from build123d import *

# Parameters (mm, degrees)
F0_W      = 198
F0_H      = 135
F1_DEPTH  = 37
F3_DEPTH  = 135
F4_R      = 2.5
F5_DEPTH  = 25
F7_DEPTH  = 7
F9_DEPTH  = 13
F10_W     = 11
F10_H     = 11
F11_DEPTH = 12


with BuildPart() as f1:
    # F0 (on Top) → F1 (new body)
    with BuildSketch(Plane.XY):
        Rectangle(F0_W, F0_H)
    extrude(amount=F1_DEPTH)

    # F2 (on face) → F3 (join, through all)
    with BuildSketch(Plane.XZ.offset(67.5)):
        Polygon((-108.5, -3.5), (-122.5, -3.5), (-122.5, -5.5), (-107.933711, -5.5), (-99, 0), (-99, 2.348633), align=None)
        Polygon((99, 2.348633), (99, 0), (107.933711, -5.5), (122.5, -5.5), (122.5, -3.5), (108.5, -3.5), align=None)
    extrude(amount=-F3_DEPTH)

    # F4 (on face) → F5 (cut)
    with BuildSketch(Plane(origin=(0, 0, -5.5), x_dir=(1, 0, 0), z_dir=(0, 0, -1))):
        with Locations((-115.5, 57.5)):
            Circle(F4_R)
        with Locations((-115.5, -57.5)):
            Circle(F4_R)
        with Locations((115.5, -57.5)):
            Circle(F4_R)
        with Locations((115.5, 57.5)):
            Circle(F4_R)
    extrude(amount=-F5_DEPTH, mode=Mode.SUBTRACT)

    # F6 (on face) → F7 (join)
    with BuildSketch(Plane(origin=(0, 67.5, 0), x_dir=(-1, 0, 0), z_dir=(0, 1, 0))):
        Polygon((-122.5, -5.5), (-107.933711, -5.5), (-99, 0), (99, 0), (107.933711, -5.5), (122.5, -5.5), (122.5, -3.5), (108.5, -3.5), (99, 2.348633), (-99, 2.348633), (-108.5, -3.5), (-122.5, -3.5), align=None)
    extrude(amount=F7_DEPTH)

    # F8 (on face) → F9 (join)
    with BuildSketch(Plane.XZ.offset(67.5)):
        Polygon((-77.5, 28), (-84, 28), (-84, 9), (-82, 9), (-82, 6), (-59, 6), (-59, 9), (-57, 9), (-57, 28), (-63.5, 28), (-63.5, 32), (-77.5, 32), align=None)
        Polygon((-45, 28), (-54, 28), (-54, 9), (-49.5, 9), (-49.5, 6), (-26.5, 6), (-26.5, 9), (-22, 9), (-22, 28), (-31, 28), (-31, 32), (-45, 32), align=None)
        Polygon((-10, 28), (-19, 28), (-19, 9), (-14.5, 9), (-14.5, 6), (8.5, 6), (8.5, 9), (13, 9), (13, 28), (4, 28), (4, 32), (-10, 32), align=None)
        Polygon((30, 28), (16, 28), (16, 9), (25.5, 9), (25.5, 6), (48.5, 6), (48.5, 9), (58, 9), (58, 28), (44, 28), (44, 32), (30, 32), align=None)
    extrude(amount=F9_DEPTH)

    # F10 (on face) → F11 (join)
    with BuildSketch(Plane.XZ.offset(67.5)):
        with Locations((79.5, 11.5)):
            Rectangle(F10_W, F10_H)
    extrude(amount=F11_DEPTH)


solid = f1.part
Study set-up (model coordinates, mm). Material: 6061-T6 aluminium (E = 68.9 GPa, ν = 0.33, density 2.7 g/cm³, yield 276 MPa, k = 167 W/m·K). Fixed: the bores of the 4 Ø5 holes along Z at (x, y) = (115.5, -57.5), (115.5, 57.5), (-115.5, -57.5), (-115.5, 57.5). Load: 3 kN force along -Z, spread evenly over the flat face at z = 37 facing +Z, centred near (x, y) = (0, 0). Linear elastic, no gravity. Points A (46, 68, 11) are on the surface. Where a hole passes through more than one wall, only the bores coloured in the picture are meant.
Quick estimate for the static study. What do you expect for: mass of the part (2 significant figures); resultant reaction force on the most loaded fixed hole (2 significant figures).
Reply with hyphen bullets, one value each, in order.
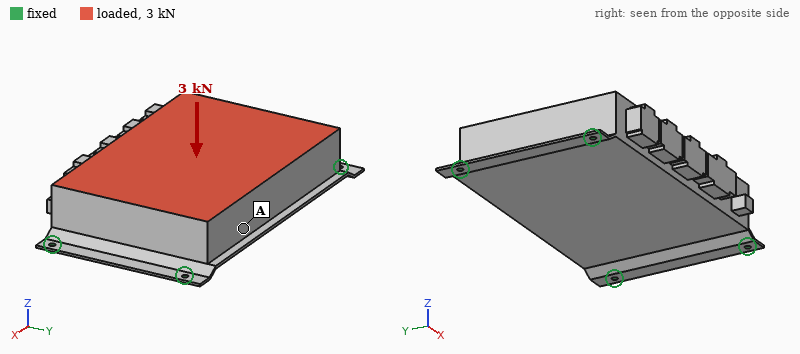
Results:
- 2.8 kg
- 1.6 kN
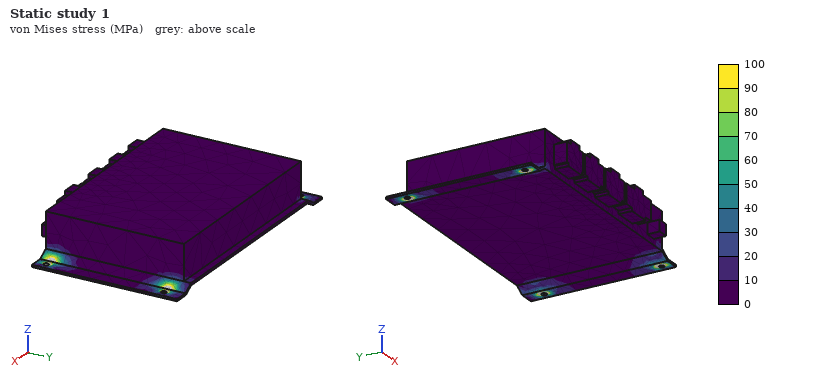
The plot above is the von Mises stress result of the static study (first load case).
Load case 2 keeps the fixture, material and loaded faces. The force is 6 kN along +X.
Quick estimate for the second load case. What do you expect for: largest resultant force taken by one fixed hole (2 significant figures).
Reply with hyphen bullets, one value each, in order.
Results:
- 1.7 kN
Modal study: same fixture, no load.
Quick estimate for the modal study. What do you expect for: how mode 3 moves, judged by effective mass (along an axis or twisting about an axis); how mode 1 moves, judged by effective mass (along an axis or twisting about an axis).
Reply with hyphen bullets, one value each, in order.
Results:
- along Y
- along Z
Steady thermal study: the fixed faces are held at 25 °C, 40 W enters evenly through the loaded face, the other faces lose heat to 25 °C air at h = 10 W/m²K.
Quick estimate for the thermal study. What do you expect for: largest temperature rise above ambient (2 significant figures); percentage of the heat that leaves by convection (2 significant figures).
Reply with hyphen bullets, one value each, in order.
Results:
- 16 K
- 28 %
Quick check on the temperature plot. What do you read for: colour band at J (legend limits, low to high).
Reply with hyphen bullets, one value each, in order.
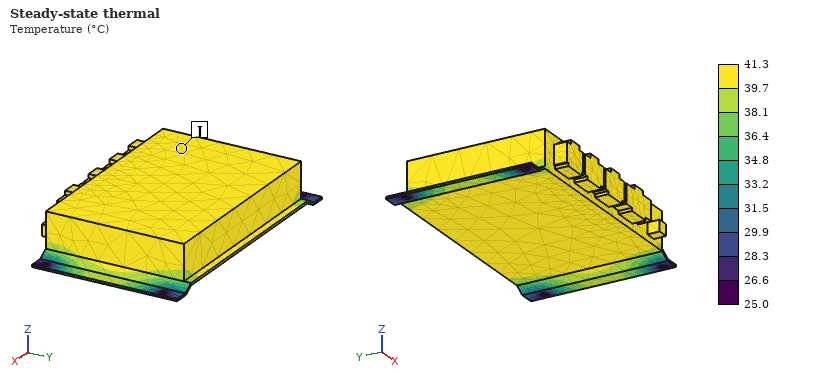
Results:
- 39.7 to 41.3 °C
